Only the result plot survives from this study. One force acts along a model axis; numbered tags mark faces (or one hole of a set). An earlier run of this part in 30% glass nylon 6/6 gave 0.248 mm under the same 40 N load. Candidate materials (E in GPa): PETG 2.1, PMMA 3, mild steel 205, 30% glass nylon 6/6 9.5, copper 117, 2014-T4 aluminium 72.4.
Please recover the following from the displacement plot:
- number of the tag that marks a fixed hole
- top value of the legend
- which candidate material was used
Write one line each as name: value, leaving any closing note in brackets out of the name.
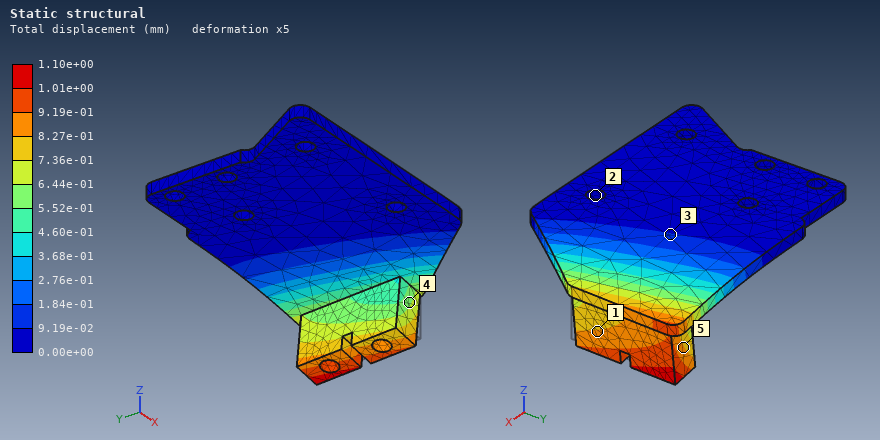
number of the tag that marks a fixed hole: 2
top value of the legend: 1.10e+00 mm
which candidate material was used: PETG
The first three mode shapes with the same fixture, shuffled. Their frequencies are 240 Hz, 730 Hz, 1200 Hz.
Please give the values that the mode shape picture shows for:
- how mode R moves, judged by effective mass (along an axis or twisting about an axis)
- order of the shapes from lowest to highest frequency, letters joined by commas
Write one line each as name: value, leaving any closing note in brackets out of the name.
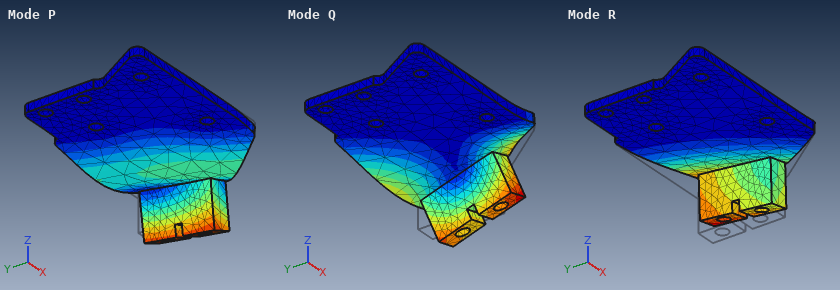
how mode R moves, judged by effective mass: along Z
order of the shapes from lowest to highest frequency, letters joined by commas: R, Q, P
